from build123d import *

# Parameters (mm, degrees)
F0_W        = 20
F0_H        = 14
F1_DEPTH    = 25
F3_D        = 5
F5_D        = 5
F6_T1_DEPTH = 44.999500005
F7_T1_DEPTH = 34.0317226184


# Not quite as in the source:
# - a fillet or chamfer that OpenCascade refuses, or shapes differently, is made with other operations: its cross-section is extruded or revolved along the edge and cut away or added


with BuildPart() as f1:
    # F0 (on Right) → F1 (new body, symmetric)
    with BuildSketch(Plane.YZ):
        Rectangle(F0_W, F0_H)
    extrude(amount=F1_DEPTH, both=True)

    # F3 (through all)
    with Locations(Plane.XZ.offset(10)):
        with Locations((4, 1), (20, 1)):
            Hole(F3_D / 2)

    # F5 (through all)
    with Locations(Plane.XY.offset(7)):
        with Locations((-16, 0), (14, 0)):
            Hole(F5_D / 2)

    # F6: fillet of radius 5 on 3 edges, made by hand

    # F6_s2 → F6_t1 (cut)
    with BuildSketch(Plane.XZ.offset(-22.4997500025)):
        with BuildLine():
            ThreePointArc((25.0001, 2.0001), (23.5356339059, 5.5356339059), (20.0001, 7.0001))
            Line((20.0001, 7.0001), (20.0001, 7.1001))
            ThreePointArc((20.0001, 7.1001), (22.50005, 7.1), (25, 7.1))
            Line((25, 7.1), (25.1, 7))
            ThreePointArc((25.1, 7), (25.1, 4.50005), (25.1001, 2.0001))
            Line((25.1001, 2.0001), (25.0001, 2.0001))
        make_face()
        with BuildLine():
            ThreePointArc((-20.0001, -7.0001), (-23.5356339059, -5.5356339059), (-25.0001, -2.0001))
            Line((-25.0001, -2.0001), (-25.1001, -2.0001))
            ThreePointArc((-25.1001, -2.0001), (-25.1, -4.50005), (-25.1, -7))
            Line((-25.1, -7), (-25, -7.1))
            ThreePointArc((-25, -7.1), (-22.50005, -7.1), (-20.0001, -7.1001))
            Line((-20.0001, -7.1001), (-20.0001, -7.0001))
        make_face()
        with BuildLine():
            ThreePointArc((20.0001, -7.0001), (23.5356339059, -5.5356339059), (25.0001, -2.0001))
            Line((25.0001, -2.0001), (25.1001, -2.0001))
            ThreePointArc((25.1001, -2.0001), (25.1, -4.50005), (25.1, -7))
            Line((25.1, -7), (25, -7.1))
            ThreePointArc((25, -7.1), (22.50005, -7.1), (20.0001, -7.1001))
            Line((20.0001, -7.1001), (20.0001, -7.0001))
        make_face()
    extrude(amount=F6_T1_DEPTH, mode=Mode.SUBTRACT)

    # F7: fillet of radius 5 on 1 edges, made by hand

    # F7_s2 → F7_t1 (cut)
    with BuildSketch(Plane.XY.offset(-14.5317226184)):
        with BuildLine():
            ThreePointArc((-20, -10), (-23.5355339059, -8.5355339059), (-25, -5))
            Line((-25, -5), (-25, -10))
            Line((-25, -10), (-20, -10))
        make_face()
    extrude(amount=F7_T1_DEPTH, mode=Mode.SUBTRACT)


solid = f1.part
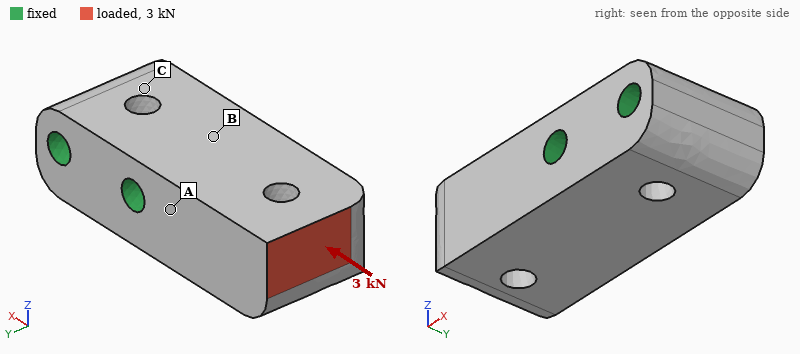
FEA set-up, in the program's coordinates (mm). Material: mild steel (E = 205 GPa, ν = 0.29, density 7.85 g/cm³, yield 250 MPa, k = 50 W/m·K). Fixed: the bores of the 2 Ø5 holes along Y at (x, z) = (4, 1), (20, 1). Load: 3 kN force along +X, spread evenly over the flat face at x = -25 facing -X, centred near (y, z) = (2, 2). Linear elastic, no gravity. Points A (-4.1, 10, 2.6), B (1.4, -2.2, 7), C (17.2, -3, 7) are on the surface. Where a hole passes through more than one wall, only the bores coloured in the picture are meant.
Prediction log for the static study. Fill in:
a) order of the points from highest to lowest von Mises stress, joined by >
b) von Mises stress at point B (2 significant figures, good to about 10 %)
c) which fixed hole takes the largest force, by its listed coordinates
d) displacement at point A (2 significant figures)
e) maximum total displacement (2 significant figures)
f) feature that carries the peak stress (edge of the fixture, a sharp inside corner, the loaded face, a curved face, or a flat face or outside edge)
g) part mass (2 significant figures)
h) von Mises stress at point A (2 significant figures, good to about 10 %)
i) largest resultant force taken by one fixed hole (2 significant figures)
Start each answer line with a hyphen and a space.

- A > B > C
- 12 MPa
- (4, 1)
- 1.0 µm
- 6.1 µm
- a curved face
- 96 g
- 26 MPa
- 2.9 kN
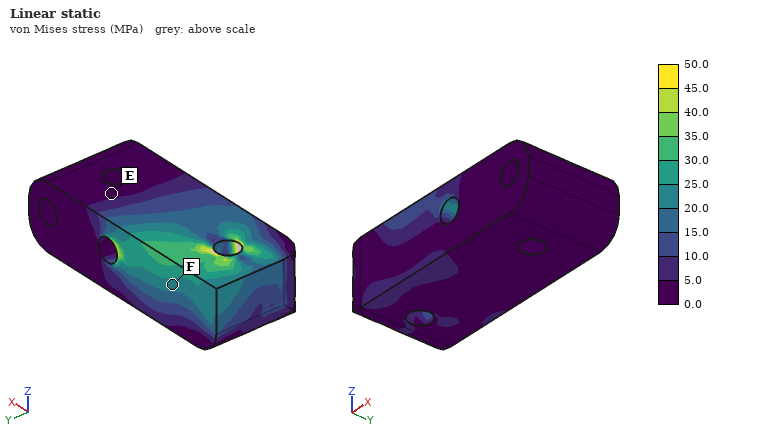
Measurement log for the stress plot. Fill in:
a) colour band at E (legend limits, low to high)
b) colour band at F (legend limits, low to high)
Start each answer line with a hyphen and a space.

- 0.0 to 5.0 MPa
- 20.0 to 25.0 MPa
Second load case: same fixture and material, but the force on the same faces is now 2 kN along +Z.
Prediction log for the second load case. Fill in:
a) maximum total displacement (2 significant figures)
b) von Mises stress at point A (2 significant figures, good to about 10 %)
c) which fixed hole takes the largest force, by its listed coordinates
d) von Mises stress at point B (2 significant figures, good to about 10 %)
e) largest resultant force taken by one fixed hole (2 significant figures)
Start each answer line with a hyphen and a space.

- 30 µm
- 32 MPa
- (4, 1)
- 69 MPa
- 3.5 kN
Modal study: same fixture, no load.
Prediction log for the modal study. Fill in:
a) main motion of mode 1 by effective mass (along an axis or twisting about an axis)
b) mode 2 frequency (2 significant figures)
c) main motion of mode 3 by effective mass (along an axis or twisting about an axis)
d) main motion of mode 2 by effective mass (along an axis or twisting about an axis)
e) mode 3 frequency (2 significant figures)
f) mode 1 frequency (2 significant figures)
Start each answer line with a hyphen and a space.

- along Z
- 16 kHz
- twisting about X
- along Y
- 25 kHz
- 11 kHz
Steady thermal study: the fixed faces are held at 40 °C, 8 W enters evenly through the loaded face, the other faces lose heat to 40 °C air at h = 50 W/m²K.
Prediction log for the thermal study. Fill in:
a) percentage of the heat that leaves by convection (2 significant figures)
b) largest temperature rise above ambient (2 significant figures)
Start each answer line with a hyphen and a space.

- 11 %
- 20 K
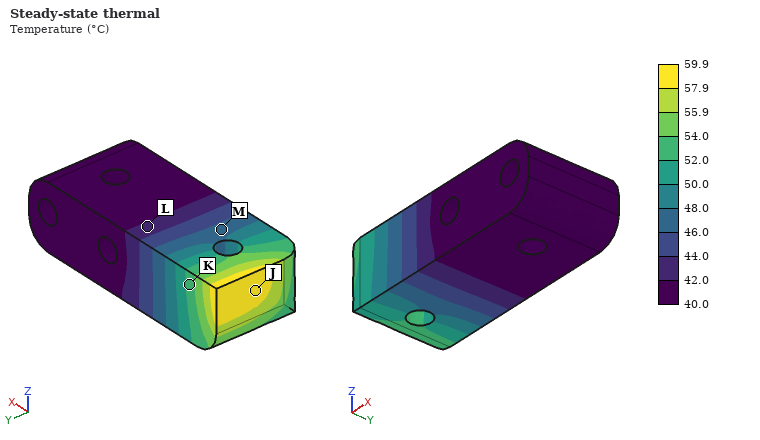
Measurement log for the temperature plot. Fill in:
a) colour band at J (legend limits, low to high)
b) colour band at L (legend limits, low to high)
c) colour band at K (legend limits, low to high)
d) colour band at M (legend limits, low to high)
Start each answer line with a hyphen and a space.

- 57.9 to 59.9 °C
- 42.0 to 44.0 °C
- 52.0 to 54.0 °C
- 46.0 to 48.0 °C
